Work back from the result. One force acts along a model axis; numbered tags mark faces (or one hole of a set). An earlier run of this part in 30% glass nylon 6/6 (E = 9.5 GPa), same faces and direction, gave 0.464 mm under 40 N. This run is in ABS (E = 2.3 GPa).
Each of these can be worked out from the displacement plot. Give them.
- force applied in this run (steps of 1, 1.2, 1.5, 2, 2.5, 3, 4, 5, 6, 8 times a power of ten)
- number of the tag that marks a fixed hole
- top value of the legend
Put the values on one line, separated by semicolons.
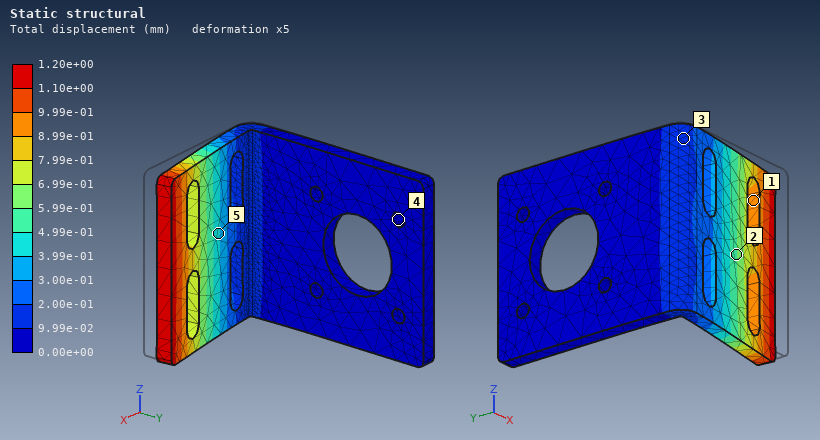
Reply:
25 N; 4; 1.20e+00 mm
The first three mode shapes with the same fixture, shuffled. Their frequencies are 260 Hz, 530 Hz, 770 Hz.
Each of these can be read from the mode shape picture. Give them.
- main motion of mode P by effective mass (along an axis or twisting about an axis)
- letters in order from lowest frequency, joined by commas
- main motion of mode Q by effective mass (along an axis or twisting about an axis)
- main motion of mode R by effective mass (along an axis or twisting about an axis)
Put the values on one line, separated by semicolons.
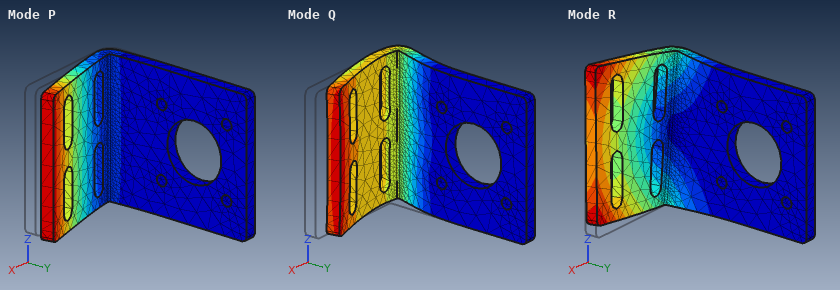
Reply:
along Y; P, R, Q; along X; along Z
